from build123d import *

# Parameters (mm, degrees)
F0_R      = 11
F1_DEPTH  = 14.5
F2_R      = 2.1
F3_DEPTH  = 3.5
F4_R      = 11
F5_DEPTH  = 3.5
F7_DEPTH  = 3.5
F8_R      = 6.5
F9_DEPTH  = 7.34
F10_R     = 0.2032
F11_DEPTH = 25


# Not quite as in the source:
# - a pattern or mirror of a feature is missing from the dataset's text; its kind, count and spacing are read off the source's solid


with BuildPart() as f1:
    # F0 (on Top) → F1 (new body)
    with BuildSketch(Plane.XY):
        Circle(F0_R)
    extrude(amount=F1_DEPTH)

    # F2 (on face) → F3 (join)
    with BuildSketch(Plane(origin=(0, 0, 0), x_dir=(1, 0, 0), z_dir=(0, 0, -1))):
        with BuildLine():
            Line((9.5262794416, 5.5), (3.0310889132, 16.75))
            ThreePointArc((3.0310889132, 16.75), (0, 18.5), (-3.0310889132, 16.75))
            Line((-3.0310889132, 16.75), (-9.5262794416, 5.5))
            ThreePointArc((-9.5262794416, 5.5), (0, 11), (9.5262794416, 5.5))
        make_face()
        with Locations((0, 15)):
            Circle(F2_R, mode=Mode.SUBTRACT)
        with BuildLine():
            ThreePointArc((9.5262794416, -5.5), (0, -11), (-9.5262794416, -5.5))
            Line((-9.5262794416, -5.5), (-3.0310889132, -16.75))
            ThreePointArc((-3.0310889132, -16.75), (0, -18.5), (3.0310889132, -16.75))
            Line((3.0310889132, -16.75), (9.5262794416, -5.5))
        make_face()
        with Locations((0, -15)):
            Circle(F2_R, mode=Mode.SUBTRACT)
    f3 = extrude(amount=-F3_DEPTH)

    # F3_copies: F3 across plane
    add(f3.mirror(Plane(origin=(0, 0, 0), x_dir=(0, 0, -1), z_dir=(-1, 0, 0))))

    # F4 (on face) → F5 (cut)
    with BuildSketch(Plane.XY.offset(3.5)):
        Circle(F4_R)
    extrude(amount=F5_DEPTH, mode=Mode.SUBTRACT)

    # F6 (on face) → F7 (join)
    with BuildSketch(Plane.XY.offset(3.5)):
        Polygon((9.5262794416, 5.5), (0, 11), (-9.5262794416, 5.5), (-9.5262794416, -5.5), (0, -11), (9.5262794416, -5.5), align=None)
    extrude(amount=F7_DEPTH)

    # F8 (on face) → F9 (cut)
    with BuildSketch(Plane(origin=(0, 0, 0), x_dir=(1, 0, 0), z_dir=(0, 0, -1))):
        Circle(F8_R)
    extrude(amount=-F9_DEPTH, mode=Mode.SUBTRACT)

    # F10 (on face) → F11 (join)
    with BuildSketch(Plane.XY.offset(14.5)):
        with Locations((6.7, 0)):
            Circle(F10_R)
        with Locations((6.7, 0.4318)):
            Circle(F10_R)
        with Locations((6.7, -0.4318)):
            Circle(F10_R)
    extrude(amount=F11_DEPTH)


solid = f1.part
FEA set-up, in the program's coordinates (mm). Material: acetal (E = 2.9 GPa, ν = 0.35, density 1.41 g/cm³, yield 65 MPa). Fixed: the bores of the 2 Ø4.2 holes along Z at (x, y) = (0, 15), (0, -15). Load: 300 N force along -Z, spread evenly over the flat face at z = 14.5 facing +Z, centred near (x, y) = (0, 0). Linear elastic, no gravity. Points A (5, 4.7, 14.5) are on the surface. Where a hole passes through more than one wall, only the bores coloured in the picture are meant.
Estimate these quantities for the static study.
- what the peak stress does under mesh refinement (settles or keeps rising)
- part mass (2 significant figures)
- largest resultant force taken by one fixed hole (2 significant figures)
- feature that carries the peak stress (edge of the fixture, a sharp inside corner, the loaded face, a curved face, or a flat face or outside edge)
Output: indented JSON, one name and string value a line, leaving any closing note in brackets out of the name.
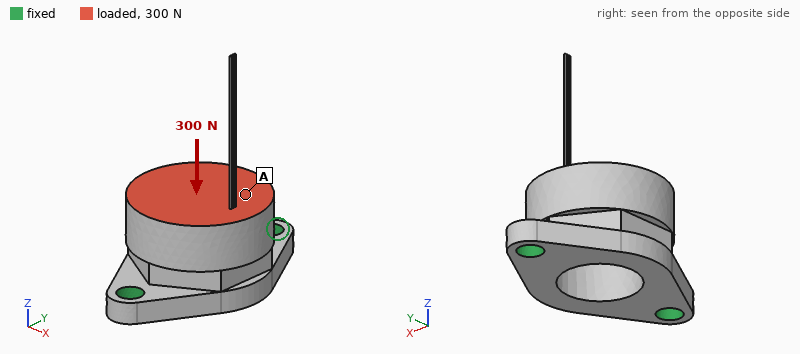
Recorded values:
{
  "what the peak stress does under mesh refinement": "keeps rising",
  "part mass": "6.7 g",
  "largest resultant force taken by one fixed hole": "170 N",
  "feature that carries the peak stress": "edge of the fixture"
}
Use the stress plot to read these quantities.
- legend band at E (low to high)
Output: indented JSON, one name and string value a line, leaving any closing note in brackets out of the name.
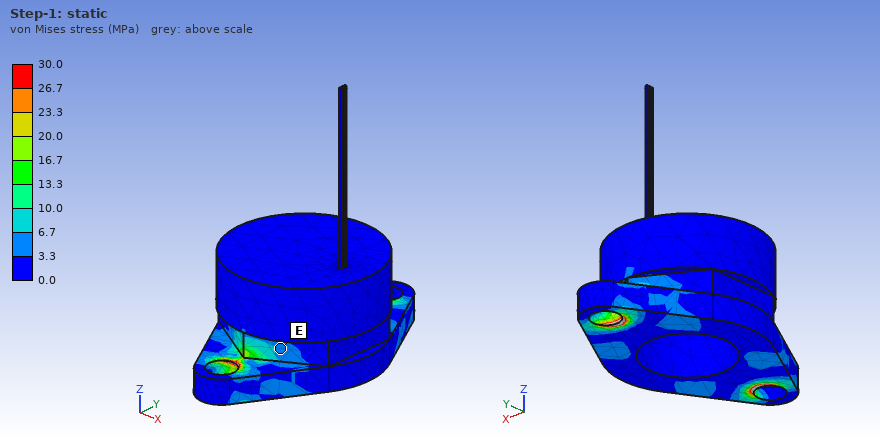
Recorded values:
{
  "legend band at E": "3.3 to 6.7 MPa"
}
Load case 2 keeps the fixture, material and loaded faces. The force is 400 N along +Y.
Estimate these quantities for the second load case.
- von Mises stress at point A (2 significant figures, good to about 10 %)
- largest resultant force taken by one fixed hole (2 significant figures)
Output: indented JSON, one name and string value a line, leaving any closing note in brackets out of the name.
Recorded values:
{
  "von Mises stress at point A": "2.4 MPa",
  "largest resultant force taken by one fixed hole": "290 N"
}
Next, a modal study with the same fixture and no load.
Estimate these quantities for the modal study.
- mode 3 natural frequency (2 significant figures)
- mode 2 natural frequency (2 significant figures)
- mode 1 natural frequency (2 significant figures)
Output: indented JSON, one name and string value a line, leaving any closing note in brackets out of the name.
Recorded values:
{
  "mode 3 natural frequency": "130 Hz",
  "mode 2 natural frequency": "130 Hz",
  "mode 1 natural frequency": "130 Hz"
}
